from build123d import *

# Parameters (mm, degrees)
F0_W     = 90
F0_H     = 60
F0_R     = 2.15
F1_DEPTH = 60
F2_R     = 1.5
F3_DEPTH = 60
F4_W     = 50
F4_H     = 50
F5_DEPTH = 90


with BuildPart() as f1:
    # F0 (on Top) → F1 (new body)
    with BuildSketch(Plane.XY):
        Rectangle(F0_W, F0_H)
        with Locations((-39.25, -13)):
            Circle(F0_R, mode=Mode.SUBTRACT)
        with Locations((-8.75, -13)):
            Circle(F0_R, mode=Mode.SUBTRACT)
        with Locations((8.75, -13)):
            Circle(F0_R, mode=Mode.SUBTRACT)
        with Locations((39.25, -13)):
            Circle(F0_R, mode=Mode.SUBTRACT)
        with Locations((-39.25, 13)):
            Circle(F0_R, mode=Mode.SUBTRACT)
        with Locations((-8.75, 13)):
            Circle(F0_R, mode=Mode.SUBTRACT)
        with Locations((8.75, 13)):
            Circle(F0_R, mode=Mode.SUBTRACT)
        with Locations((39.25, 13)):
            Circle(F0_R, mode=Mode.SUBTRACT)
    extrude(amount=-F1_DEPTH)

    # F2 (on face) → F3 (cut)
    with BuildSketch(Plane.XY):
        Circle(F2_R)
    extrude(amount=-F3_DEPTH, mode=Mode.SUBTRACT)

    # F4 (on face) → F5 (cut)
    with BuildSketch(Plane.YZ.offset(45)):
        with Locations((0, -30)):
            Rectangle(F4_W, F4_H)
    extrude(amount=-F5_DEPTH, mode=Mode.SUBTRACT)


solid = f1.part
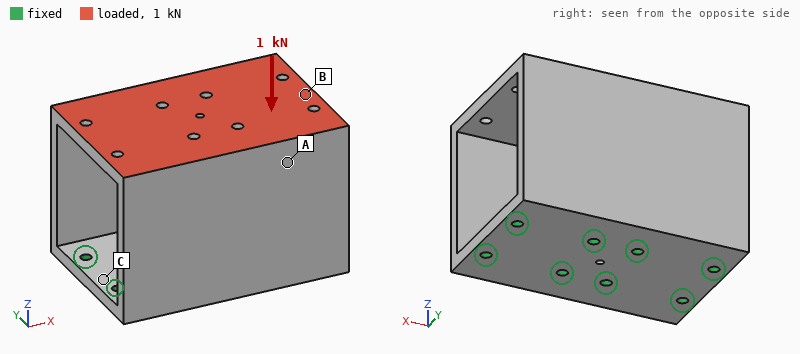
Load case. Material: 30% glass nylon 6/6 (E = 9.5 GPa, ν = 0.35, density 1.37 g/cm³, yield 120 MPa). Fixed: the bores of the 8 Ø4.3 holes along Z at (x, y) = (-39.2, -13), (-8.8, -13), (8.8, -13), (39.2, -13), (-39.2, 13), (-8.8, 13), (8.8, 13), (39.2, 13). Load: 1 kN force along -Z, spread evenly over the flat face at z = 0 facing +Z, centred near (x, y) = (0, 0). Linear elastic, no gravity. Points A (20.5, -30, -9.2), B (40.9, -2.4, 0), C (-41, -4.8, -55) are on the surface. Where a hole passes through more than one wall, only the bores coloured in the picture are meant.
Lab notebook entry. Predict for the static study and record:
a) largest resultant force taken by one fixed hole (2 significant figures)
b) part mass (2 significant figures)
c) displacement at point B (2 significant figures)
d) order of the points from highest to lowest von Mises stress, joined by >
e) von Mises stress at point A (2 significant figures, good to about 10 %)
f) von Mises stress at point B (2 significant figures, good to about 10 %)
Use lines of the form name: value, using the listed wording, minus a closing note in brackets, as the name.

largest resultant force taken by one fixed hole: 140 N
part mass: 130 g
displacement at point B: 0.18 mm
order of the points from highest to lowest von Mises stress, joined by >: B > A > C
von Mises stress at point A: 4.4 MPa
von Mises stress at point B: 9.7 MPa
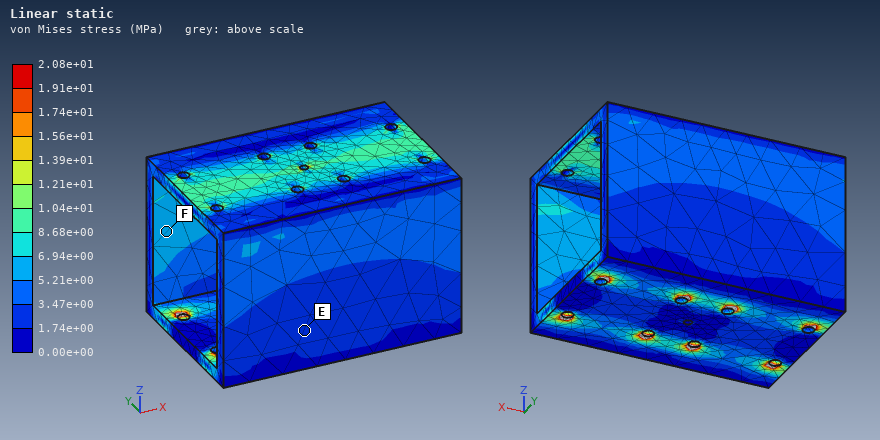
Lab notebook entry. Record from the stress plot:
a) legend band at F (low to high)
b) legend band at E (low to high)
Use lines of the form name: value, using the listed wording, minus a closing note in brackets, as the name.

legend band at F: 5.21e+00 to 6.94e+00 MPa
legend band at E: 1.74e+00 to 3.47e+00 MPa
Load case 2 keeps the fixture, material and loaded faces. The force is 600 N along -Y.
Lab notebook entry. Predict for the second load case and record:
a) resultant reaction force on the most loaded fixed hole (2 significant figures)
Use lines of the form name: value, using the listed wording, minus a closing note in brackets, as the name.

resultant reaction force on the most loaded fixed hole: 190 N
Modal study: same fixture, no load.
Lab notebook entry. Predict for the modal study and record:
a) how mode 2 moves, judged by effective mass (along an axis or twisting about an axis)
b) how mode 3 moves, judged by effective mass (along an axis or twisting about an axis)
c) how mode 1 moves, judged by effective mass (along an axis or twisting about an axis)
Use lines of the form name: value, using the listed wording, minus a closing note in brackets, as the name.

how mode 2 moves, judged by effective mass: along X
how mode 3 moves, judged by effective mass: twisting about Z
how mode 1 moves, judged by effective mass: along Y
